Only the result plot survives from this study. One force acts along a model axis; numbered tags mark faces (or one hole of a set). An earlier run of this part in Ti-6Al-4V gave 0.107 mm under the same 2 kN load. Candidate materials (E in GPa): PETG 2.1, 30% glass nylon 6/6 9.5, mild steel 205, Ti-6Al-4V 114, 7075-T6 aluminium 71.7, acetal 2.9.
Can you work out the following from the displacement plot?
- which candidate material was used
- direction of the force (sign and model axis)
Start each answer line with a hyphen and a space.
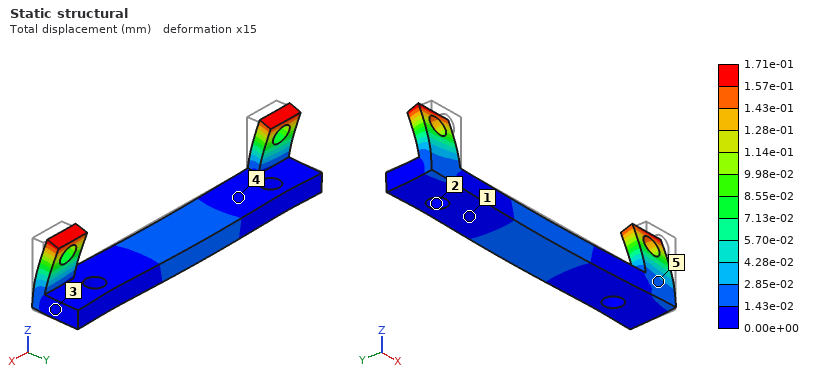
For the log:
- 7075-T6 aluminium
- +Y
